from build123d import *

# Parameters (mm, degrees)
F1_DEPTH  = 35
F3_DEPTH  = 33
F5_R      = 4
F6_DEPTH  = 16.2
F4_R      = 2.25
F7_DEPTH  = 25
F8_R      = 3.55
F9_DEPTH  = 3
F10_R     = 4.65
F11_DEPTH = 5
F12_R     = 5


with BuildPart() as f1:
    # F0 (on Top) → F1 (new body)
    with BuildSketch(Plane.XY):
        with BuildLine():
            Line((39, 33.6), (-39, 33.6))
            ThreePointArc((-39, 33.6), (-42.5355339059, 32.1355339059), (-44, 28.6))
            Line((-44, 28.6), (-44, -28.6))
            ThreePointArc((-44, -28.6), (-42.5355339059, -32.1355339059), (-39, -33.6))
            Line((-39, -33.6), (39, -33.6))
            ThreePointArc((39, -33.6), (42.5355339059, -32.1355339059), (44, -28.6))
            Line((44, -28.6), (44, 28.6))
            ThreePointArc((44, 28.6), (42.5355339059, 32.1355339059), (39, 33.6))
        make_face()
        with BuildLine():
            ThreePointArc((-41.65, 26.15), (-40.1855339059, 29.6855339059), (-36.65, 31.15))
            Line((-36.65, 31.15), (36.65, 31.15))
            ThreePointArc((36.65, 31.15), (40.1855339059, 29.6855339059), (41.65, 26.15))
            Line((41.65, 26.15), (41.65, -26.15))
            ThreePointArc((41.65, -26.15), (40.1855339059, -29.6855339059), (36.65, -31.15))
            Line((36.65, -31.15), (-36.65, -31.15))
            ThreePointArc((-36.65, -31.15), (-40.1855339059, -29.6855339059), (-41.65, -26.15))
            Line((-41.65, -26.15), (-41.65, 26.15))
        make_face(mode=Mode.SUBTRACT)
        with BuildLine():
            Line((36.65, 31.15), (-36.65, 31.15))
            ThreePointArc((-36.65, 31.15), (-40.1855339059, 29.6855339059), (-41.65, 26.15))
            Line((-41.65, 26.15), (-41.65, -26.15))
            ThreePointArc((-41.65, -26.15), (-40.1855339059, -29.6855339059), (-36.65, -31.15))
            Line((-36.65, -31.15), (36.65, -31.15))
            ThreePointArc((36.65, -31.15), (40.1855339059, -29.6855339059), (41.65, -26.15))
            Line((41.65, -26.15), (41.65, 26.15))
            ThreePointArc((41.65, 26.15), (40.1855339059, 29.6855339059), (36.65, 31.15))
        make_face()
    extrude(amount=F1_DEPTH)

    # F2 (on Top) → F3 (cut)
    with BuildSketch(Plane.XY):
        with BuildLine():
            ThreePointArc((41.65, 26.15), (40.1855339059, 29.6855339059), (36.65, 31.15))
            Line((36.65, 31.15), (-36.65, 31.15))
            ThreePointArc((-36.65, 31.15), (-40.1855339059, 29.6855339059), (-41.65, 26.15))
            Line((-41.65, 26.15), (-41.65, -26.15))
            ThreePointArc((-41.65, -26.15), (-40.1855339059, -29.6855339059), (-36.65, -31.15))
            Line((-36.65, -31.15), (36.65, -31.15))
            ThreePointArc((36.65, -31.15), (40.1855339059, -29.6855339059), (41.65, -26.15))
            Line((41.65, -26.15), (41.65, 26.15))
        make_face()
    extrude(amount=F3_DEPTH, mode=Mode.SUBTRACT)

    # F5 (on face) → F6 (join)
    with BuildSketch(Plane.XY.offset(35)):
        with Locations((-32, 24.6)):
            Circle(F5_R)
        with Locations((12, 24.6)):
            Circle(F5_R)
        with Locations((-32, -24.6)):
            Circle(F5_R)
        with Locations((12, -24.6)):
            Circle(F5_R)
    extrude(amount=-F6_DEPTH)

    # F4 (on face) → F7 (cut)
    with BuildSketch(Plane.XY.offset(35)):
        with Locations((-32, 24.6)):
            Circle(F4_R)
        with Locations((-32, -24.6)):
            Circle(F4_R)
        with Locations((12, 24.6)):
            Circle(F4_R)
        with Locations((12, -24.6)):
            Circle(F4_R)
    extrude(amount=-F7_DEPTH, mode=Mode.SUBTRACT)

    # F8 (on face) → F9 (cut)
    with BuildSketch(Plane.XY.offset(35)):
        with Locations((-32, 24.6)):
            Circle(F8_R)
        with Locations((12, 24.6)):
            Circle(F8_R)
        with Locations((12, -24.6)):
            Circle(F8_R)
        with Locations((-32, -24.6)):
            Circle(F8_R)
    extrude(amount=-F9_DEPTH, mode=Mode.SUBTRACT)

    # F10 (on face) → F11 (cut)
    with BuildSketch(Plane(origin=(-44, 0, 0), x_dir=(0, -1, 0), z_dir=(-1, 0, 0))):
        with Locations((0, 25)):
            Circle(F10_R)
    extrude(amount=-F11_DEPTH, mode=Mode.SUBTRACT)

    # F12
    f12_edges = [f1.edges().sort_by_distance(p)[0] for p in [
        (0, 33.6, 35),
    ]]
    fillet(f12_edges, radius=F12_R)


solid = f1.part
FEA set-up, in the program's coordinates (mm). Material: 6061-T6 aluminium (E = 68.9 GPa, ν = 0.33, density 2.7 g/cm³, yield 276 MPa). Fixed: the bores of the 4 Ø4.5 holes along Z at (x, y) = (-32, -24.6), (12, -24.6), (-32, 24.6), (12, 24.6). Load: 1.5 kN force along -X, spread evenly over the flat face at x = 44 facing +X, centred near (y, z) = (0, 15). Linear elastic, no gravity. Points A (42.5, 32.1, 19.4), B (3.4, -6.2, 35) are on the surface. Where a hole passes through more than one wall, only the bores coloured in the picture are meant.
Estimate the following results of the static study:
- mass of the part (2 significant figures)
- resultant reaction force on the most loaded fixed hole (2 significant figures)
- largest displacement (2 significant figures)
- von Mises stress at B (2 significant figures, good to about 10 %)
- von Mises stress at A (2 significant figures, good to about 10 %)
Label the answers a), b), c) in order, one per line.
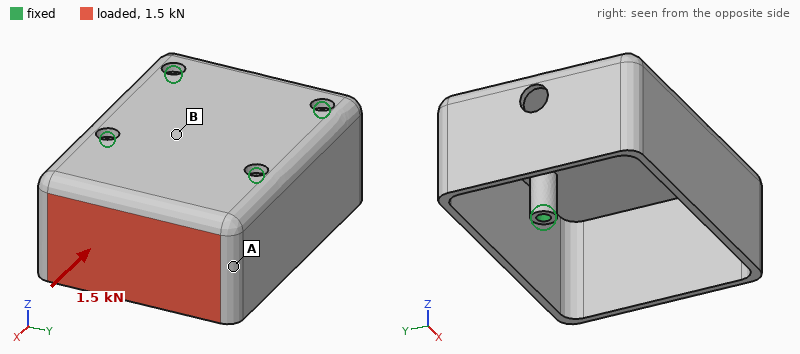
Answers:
a) 96 g
b) 480 N
c) 0.70 mm
d) 13 MPa
e) 88 MPa
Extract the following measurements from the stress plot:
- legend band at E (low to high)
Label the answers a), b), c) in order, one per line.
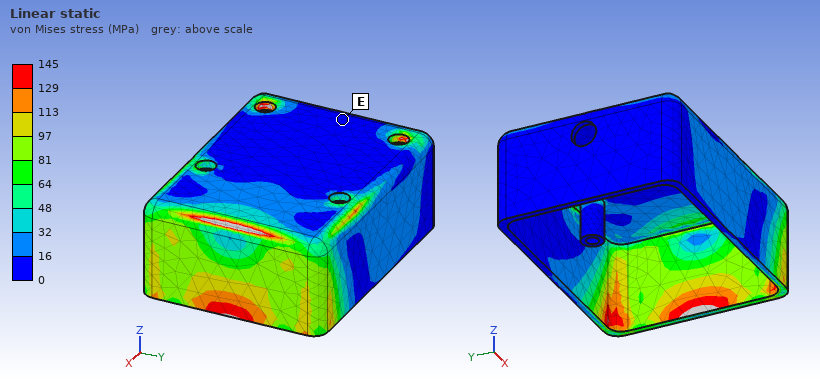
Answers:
a) 0 to 16 MPa
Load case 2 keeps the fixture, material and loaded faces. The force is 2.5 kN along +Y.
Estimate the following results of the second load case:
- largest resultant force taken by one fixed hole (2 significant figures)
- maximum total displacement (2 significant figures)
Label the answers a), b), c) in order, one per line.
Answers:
a) 2.1 kN
b) 0.43 mm
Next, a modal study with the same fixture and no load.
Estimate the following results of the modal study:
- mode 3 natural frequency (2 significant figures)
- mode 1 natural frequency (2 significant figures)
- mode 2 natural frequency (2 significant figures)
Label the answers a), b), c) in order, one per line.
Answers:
a) 2400 Hz
b) 1900 Hz
c) 1900 Hz
